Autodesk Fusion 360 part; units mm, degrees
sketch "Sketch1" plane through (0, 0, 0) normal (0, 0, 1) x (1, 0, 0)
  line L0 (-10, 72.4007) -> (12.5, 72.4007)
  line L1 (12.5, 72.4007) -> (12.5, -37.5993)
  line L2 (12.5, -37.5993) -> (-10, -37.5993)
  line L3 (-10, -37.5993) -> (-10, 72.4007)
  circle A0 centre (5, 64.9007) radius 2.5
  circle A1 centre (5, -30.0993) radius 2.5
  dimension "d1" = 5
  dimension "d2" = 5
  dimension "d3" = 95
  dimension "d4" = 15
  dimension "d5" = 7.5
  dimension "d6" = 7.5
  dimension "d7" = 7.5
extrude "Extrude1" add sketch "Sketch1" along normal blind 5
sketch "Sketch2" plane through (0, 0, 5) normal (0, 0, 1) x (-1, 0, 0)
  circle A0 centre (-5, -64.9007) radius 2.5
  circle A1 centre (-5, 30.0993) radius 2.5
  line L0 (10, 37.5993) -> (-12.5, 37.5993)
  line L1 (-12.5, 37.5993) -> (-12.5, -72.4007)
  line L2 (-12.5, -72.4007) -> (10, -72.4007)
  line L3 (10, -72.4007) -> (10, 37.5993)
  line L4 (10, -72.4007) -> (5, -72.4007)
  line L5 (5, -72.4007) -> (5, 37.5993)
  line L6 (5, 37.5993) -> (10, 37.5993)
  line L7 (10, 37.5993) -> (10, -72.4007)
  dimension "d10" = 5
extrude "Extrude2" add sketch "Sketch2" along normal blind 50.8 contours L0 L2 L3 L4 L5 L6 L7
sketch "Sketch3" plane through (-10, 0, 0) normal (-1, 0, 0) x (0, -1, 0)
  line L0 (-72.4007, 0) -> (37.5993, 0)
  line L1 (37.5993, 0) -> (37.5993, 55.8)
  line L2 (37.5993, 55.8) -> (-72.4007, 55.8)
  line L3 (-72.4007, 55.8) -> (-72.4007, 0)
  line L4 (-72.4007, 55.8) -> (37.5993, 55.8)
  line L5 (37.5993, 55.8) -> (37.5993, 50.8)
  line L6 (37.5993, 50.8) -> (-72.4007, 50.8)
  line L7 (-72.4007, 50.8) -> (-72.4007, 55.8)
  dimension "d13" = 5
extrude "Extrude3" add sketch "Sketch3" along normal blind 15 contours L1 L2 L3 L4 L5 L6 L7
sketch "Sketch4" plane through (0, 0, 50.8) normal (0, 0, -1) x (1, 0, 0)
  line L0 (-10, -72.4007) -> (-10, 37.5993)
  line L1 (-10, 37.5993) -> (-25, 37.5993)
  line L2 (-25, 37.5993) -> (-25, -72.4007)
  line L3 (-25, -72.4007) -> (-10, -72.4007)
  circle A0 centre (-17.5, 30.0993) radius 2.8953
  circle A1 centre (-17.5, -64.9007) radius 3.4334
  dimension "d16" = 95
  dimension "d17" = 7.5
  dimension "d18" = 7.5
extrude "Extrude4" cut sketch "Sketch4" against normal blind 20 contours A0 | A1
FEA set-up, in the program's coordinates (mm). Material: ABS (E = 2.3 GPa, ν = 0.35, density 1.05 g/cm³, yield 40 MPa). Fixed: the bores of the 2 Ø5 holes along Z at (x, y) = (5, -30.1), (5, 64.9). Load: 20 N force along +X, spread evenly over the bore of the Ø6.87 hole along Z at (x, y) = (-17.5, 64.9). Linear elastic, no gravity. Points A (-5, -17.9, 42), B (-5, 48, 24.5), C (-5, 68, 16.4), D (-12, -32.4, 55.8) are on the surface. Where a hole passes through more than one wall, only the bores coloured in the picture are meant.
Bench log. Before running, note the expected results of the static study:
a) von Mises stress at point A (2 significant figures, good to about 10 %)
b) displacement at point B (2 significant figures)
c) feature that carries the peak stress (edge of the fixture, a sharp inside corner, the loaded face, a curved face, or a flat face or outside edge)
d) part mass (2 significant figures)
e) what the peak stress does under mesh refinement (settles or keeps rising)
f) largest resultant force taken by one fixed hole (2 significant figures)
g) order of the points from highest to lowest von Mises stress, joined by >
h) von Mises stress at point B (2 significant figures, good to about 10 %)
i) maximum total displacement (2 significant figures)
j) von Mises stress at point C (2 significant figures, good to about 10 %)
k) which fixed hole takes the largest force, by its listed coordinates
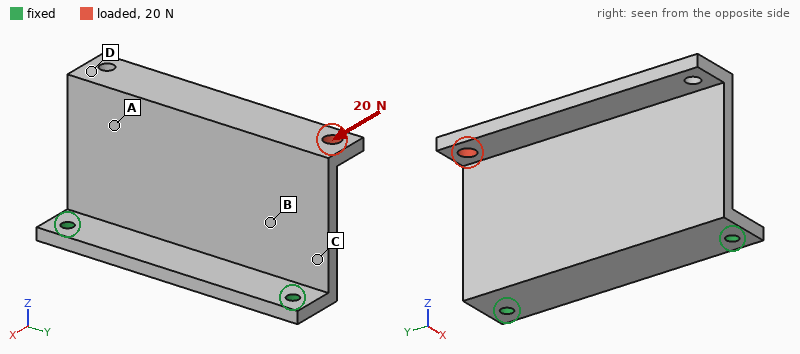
0.95 MPa
0.36 mm
edge of the fixture
50 g
keeps rising
21 N
C > B > A > D
1.9 MPa
1.3 mm
2.7 MPa
(5, 64.9)
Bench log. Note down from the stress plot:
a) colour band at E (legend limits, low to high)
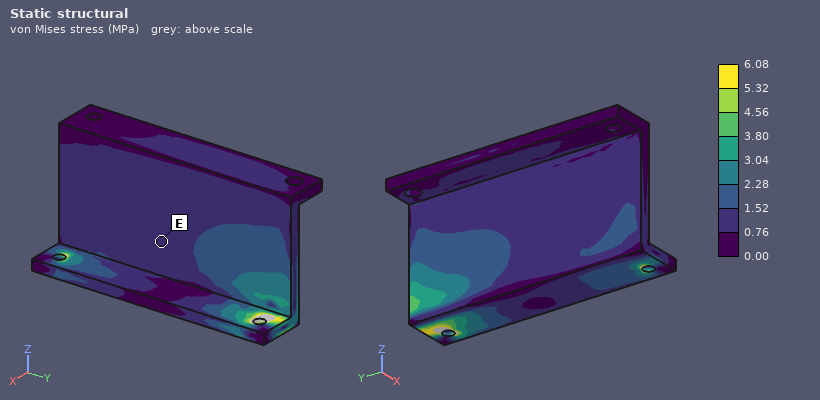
0.76 to 1.52 MPa
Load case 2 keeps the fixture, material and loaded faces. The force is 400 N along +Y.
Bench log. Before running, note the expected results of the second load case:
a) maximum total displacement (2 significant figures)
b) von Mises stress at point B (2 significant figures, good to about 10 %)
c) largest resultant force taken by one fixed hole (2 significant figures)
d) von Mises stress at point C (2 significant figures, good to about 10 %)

1.2 mm
3.2 MPa
310 N
8.5 MPa
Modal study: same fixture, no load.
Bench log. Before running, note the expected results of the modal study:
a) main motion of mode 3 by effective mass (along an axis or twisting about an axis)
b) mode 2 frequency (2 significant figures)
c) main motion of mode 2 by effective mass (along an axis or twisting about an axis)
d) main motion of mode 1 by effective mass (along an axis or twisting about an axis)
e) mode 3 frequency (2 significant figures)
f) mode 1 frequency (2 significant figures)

along Y
420 Hz
twisting about Z
along X
1100 Hz
180 Hz
